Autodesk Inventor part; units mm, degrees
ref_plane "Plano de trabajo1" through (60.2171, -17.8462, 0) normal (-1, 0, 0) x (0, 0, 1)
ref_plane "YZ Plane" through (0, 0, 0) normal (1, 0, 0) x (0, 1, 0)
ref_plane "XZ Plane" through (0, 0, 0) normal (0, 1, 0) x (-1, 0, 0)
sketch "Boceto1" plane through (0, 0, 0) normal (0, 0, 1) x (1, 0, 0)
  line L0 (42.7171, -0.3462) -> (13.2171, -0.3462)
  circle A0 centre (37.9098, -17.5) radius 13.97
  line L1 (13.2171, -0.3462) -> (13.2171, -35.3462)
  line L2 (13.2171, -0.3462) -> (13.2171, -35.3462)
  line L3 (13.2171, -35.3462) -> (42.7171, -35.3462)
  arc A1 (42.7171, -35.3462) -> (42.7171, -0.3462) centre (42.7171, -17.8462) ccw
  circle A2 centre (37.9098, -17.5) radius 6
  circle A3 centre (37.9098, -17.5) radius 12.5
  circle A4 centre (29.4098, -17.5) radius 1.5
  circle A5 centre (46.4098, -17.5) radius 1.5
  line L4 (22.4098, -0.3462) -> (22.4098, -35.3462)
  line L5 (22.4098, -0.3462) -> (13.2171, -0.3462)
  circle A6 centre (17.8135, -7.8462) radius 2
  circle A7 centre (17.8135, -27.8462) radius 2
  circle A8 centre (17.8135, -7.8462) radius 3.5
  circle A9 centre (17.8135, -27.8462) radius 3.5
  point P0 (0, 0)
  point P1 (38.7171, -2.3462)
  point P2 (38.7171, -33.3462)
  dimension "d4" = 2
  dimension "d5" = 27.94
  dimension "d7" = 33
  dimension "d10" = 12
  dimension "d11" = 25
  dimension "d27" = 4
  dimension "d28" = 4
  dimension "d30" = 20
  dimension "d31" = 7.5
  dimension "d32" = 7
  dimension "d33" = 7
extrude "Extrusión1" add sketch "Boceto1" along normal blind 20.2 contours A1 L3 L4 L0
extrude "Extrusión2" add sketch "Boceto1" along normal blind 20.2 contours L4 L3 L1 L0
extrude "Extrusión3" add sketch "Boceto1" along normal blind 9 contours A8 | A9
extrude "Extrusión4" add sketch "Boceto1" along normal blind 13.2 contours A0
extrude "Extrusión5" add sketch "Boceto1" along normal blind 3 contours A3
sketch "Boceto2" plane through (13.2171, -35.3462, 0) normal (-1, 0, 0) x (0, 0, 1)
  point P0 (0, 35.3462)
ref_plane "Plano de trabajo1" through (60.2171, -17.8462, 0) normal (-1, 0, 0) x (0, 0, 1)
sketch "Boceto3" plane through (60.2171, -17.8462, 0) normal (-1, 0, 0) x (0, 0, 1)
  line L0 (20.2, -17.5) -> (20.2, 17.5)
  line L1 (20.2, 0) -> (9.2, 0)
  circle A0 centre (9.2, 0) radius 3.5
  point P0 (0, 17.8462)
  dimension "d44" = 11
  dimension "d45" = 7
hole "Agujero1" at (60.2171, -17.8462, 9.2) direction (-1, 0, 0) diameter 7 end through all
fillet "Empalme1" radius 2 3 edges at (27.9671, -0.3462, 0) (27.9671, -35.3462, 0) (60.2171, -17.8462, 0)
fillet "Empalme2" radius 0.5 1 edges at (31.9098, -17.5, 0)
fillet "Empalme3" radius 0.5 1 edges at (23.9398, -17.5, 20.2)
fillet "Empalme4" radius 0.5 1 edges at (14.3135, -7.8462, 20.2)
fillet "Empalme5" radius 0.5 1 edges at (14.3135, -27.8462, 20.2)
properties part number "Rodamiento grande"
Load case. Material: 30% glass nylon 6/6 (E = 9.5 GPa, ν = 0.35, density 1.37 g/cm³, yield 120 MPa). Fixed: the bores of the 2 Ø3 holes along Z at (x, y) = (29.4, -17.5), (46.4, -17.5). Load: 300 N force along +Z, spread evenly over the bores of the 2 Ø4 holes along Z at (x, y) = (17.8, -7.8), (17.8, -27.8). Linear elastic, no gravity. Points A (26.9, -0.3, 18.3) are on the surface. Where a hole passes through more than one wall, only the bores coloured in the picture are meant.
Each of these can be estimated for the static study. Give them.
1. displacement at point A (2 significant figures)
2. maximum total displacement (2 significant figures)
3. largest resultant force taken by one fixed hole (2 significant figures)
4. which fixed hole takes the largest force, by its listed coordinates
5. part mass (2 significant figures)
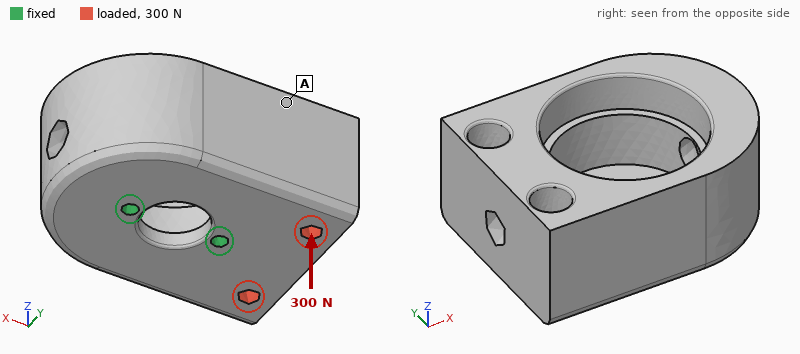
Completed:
56 µm
98 µm
420 N
(29.4, -17.5)
26 g
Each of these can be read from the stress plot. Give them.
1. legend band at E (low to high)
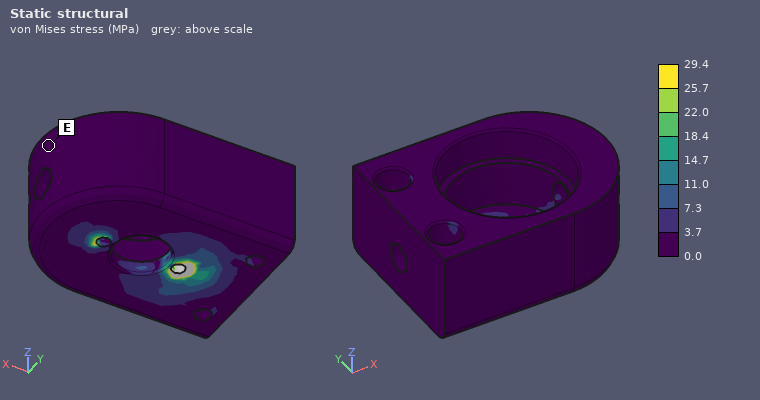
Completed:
0.0 to 3.7 MPa
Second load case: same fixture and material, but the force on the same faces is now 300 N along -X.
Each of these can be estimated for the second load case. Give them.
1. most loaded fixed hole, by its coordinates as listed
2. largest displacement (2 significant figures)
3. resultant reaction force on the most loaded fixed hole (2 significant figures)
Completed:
(29.4, -17.5)
20 µm
200 N
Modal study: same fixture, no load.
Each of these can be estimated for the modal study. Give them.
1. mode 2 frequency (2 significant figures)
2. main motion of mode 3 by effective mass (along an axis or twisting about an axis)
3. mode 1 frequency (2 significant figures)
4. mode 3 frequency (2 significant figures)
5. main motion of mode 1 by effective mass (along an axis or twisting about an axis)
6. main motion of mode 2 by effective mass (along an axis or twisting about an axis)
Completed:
2600 Hz
twisting about Z
1200 Hz
3900 Hz
along Y
along X
